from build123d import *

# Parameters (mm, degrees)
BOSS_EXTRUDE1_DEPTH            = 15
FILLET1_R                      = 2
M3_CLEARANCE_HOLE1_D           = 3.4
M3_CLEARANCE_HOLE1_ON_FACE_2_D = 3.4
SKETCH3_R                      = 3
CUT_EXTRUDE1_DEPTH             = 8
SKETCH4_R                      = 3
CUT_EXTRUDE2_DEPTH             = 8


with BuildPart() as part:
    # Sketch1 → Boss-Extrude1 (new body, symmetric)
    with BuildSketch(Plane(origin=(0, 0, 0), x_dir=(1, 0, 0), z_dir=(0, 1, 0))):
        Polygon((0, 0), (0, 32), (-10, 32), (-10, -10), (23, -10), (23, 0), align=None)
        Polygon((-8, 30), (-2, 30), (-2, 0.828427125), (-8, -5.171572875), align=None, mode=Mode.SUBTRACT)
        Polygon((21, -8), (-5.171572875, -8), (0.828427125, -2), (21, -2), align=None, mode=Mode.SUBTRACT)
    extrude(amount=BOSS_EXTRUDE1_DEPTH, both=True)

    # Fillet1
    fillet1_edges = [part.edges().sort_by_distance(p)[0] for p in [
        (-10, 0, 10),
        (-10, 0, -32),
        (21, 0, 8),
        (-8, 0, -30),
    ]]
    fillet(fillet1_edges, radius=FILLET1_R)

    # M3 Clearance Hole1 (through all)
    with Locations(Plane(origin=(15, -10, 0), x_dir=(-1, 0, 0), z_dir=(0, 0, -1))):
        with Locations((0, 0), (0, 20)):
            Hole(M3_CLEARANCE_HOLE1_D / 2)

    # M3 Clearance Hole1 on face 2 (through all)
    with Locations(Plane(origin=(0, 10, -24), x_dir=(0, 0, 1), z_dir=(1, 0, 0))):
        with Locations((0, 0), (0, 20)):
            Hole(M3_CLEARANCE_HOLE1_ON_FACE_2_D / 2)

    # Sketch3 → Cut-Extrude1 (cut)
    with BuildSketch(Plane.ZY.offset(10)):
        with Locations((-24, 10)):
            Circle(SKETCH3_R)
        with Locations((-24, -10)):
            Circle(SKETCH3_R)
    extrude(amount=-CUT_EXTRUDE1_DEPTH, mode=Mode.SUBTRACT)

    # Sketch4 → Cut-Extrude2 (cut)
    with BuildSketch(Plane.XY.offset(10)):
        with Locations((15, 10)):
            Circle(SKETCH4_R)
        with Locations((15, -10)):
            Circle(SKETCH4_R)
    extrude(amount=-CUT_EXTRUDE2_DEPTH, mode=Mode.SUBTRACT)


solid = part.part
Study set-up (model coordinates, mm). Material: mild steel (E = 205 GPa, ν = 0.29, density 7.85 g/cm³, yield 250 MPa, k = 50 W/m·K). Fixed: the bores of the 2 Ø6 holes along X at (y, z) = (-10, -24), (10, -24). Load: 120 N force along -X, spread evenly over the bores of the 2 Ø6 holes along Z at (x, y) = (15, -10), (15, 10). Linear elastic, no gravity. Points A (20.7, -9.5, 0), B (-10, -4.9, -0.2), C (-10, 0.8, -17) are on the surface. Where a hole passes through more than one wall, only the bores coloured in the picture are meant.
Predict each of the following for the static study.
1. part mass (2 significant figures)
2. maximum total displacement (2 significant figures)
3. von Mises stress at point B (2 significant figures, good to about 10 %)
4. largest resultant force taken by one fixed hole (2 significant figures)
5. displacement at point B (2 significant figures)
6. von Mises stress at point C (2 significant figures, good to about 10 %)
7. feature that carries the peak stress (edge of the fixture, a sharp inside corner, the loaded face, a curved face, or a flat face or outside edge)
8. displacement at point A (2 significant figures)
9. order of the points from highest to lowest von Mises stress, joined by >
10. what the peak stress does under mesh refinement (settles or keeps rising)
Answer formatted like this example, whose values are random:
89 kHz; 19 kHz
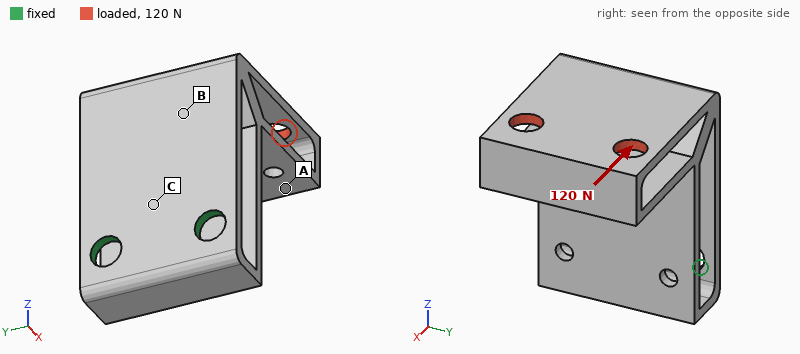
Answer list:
73 g; 0.12 mm; 21 MPa; 62 N; 0.066 mm; 63 MPa; edge of the fixture; 0.099 mm; C > B > A; keeps rising
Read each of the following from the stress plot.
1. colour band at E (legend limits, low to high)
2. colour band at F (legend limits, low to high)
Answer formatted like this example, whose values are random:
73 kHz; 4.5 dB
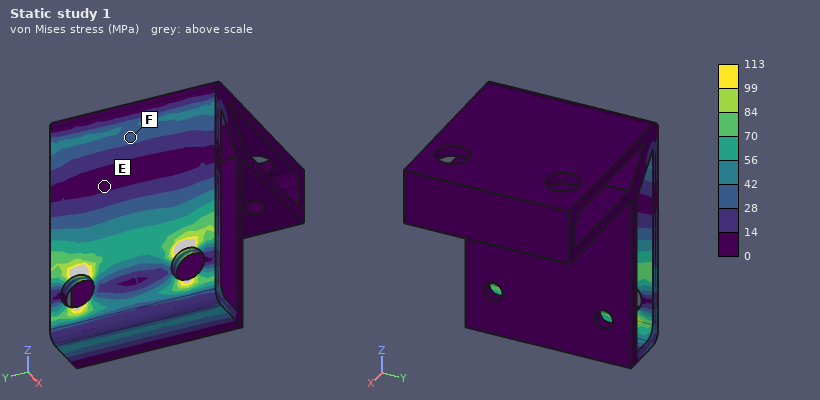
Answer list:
0 to 14 MPa; 28 to 42 MPa
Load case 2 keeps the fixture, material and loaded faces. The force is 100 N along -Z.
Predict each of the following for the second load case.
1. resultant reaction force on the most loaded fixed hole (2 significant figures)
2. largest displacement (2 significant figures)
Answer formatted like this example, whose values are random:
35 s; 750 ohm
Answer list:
51 N; 85 µm
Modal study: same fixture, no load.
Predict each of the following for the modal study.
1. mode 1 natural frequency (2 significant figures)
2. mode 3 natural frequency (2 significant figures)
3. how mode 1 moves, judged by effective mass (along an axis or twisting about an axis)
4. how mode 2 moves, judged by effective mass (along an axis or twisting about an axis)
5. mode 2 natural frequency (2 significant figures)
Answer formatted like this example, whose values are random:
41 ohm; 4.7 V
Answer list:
840 Hz; 2200 Hz; along X; along Y; 1600 Hz
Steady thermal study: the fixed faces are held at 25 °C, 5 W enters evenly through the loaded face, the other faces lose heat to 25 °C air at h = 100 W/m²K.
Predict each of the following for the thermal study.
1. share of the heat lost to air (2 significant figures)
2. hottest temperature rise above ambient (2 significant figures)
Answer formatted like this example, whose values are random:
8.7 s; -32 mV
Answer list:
90 %; 20 K
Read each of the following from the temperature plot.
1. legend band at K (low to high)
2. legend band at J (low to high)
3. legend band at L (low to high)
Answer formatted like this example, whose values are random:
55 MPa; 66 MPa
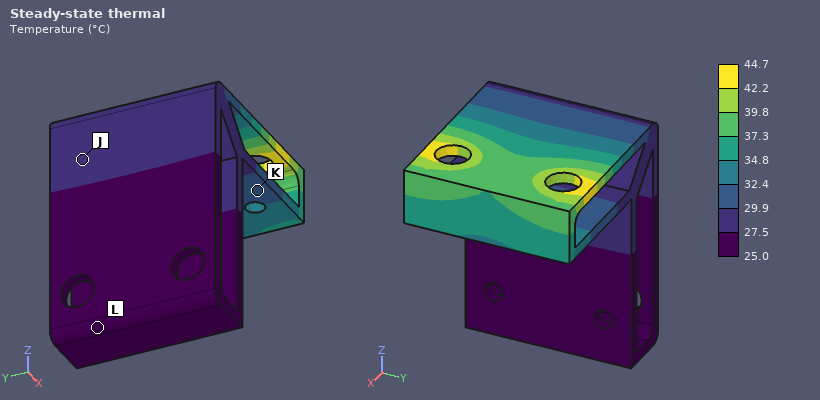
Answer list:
29.9 to 32.4 °C; 27.5 to 29.9 °C; 25.0 to 27.5 °C
